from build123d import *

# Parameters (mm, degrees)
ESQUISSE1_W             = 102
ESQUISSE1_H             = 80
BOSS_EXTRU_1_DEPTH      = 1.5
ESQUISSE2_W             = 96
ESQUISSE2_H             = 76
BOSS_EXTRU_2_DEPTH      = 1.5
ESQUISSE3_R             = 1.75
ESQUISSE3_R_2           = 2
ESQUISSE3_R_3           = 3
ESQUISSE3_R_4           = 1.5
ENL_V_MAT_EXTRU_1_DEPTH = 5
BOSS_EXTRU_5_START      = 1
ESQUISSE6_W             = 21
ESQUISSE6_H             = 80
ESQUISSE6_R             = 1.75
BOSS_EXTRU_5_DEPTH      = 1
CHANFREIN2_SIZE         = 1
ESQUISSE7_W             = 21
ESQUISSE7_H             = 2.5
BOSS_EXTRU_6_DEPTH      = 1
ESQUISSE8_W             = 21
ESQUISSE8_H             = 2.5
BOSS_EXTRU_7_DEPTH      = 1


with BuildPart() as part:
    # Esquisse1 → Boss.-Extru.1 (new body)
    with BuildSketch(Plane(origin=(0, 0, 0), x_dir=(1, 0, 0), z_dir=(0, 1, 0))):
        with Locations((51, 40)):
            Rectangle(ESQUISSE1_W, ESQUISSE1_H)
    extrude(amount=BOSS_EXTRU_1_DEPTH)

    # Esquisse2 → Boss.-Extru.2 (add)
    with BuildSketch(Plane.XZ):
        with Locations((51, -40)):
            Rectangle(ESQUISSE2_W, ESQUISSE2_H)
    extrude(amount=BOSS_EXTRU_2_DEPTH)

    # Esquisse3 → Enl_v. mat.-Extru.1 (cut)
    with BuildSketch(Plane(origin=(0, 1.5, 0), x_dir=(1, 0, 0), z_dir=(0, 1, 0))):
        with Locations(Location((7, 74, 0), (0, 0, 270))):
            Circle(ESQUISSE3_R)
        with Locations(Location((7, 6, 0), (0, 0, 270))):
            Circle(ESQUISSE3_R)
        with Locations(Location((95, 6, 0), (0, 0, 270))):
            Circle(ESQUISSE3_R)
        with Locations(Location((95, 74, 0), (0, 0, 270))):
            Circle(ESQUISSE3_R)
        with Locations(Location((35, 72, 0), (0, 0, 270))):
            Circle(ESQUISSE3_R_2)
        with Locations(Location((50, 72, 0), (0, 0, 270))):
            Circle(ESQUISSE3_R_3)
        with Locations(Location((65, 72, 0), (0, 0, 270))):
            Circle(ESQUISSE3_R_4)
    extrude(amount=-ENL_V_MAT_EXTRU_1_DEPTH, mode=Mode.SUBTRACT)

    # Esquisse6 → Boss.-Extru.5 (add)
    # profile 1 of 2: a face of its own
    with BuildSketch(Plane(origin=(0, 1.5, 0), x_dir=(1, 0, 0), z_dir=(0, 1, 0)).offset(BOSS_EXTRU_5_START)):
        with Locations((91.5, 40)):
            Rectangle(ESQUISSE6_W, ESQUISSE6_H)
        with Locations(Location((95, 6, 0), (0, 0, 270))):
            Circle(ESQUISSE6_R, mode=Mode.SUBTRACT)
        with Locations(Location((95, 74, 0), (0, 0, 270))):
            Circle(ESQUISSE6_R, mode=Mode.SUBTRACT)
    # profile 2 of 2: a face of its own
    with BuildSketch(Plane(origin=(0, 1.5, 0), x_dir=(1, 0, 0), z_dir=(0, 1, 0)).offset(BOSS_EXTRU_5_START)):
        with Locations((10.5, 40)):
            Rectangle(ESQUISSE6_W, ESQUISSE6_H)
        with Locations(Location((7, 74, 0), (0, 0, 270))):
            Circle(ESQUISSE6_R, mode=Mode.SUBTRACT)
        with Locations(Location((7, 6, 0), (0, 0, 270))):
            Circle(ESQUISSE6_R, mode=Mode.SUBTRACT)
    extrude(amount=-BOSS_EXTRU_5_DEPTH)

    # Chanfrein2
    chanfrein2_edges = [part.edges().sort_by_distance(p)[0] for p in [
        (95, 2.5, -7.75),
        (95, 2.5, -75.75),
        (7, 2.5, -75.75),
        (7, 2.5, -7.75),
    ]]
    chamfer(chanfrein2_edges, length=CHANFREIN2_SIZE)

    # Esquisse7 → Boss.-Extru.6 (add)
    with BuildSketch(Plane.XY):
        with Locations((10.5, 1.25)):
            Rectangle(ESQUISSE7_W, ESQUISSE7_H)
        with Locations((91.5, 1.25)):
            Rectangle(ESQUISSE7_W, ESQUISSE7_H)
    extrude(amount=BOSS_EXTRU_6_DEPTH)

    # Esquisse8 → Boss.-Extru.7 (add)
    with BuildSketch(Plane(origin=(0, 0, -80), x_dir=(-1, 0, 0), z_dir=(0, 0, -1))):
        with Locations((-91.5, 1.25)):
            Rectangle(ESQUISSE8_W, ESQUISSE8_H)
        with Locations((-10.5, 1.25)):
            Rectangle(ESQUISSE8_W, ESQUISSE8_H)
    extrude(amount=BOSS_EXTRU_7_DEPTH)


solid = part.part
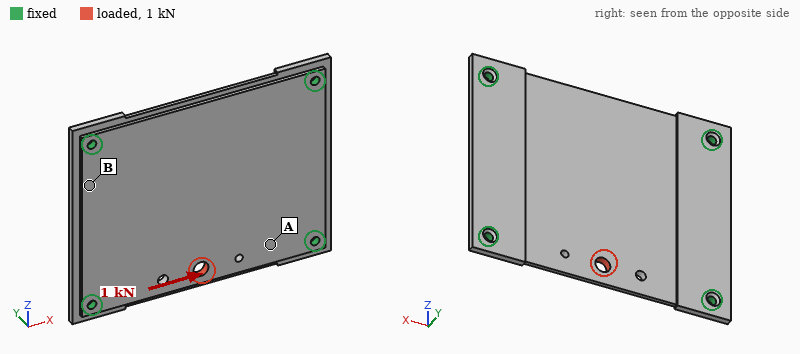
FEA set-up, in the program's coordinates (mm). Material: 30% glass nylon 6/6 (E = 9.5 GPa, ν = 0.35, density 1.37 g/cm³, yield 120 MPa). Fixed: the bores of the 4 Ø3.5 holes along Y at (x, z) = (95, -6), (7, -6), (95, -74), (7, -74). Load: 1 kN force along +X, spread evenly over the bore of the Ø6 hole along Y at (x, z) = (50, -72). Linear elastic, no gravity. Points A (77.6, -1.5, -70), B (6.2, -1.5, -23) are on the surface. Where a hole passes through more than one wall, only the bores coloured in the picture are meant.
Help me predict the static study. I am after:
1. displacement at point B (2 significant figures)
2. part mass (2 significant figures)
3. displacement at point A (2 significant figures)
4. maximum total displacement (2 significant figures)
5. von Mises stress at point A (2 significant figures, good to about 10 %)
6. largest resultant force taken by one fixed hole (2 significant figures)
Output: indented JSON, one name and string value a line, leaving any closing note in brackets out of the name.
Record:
{
  "displacement at point B": "8.4 µm",
  "part mass": "36 g",
  "displacement at point A": "19 µm",
  "maximum total displacement": "50 µm",
  "von Mises stress at point A": "5.1 MPa",
  "largest resultant force taken by one fixed hole": "390 N"
}
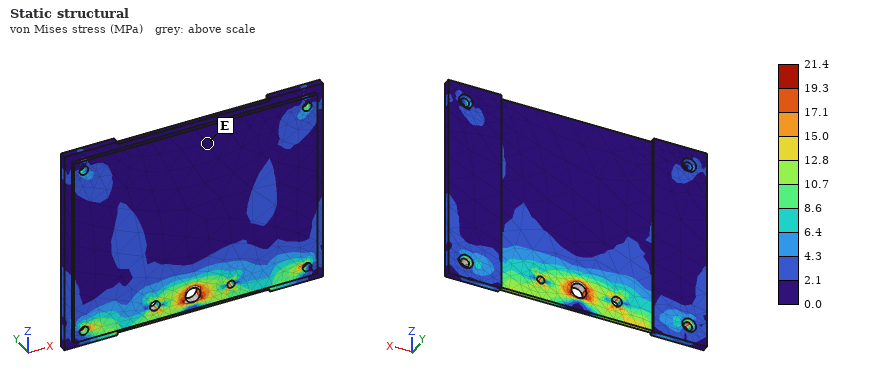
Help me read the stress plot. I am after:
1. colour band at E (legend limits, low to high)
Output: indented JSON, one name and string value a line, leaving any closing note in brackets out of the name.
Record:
{
  "colour band at E": "0.0 to 2.1 MPa"
}
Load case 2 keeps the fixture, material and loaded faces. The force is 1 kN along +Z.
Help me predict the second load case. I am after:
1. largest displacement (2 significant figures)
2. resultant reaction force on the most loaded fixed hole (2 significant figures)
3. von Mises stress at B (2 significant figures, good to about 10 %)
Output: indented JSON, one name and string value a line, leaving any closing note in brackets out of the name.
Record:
{
  "largest displacement": "81 µm",
  "resultant reaction force on the most loaded fixed hole": "310 N",
  "von Mises stress at B": "3.0 MPa"
}
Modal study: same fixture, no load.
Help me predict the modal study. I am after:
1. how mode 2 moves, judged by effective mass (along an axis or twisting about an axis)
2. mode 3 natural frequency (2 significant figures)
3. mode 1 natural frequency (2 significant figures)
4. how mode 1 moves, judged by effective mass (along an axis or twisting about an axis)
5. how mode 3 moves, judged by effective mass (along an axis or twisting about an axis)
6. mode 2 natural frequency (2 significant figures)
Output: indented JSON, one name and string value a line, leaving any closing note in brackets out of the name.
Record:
{
  "how mode 2 moves, judged by effective mass": "twisting about X",
  "mode 3 natural frequency": "1900 Hz",
  "mode 1 natural frequency": "930 Hz",
  "how mode 1 moves, judged by effective mass": "along Y",
  "how mode 3 moves, judged by effective mass": "twisting about Z",
  "mode 2 natural frequency": "1500 Hz"
}
